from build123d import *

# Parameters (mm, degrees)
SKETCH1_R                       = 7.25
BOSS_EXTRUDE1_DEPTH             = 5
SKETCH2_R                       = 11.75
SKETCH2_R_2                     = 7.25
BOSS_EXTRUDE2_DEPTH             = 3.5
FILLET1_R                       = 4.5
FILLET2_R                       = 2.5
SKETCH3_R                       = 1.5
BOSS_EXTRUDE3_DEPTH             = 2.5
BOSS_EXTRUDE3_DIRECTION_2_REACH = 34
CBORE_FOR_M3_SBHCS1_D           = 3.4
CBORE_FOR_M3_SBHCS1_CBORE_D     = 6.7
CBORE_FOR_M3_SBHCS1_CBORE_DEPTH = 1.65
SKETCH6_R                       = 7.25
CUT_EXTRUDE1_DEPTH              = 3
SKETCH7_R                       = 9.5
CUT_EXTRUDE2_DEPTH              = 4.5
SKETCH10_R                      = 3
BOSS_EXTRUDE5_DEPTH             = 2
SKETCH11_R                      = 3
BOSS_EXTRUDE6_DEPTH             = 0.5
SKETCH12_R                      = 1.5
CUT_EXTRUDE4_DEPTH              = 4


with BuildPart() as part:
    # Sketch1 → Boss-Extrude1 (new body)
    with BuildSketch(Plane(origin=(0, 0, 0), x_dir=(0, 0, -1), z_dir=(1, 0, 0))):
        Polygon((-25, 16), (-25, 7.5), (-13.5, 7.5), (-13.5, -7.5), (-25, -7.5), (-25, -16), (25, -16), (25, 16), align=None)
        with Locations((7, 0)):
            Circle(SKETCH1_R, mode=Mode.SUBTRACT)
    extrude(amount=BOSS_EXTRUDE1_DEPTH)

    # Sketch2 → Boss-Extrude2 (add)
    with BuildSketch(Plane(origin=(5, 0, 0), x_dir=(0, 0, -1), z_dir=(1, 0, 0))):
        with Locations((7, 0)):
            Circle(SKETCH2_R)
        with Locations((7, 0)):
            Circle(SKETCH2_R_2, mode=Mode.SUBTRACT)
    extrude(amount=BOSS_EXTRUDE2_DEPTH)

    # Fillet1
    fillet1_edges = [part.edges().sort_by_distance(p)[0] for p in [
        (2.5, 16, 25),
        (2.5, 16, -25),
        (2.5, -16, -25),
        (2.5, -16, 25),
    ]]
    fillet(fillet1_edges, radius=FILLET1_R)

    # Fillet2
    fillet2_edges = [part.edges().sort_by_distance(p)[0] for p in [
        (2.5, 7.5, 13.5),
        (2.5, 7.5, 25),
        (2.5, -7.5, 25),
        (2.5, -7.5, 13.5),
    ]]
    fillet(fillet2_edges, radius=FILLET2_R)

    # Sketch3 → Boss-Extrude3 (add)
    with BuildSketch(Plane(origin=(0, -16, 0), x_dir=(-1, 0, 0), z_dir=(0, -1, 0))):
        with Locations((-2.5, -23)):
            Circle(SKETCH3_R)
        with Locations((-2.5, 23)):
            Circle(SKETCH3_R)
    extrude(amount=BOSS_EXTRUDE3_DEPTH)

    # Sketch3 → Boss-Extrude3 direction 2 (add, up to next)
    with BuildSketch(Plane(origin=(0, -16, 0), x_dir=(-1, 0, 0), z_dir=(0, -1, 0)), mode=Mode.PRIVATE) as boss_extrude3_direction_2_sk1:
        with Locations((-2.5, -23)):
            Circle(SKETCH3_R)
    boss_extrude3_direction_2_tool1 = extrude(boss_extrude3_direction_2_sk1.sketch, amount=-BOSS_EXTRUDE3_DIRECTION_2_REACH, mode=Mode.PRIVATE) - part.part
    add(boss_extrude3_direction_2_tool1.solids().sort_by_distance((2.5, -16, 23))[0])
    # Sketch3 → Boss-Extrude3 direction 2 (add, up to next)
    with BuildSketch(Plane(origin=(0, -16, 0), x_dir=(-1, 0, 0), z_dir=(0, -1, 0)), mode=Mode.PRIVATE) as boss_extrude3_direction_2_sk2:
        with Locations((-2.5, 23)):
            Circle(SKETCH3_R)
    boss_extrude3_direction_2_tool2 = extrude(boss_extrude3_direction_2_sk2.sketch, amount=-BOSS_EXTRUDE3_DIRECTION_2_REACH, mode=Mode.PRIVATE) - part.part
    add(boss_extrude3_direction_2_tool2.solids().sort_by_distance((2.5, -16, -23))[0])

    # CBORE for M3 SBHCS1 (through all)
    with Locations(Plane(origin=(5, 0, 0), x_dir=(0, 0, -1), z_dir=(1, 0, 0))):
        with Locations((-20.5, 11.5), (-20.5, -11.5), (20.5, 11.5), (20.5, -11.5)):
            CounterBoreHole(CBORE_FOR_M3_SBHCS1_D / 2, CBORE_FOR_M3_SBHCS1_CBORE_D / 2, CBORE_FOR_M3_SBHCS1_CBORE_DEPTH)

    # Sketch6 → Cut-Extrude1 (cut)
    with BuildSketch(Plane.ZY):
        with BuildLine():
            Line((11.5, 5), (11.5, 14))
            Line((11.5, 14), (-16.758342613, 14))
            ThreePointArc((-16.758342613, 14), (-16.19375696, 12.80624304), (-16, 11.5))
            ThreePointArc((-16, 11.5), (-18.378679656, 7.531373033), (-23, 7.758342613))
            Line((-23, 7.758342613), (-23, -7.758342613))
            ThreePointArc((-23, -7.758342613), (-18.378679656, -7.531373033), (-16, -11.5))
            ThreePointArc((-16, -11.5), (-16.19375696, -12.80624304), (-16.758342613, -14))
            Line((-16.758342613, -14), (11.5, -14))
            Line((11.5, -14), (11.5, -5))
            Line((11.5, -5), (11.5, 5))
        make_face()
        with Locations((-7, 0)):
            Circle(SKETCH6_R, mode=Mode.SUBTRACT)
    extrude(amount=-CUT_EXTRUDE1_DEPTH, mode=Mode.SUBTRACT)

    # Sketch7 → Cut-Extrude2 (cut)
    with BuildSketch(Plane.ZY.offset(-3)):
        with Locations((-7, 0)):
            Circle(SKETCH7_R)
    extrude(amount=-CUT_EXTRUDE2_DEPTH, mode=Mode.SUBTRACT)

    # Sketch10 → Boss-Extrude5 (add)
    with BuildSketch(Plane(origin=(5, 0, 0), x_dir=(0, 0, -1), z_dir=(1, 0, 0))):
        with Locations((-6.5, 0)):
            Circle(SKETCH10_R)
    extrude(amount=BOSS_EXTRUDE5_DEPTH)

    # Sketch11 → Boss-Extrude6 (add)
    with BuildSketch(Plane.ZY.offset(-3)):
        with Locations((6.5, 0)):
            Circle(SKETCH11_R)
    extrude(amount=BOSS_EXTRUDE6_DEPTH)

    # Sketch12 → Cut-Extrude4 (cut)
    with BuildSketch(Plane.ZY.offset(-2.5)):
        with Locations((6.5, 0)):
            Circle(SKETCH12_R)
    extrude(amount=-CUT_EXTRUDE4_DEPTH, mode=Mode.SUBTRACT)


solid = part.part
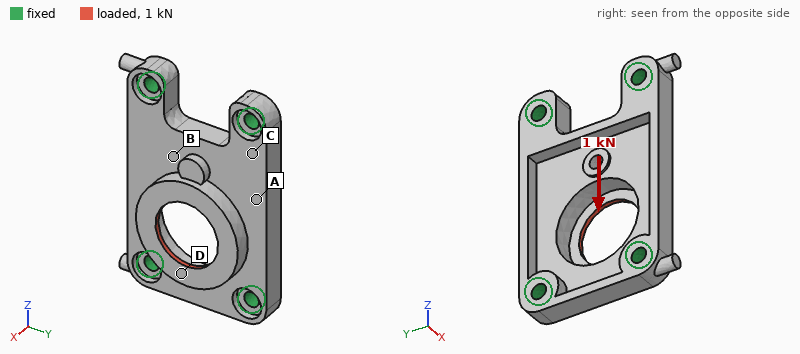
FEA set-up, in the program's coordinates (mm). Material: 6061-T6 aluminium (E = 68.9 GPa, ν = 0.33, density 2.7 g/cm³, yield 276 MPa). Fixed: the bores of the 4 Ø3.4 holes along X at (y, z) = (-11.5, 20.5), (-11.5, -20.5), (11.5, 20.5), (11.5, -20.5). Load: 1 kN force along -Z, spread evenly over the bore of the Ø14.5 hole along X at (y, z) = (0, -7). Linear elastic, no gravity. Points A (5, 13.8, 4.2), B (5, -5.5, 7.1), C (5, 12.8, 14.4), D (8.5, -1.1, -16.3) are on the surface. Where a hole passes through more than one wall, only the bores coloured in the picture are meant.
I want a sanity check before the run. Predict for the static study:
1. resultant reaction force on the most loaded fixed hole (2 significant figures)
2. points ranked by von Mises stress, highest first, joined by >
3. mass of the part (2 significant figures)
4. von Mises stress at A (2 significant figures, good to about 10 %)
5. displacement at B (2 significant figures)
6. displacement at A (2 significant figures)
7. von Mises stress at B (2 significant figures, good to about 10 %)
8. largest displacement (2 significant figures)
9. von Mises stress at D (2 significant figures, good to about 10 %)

270 N
D > B > A > C
11 g
13 MPa
5.7 µm
5.4 µm
17 MPa
14 µm
34 MPa
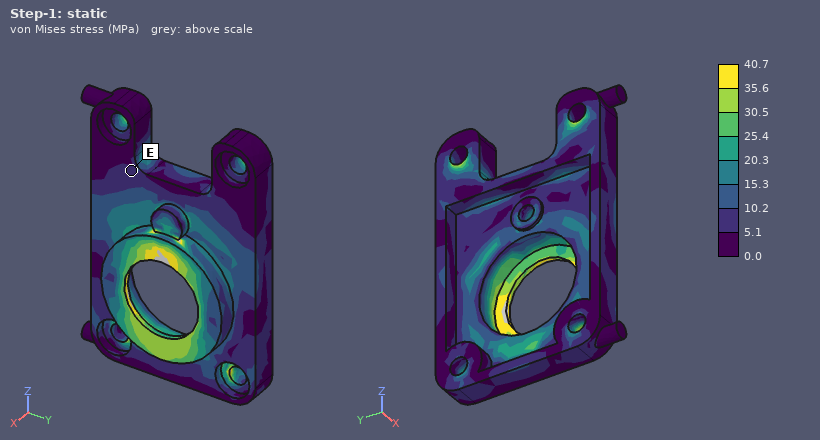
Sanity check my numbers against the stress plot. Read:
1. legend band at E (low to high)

5.1 to 10.2 MPa
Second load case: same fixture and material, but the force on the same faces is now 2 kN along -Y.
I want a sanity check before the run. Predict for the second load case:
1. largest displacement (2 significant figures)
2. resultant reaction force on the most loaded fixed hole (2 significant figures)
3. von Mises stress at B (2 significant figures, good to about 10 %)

31 µm
760 N
42 MPa
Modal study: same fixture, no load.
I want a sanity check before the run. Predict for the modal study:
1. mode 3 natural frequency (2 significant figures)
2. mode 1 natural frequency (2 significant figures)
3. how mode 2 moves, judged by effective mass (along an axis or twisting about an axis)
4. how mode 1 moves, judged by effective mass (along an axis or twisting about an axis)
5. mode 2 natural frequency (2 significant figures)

21 kHz
12 kHz
twisting about Z
along X
15 kHz
